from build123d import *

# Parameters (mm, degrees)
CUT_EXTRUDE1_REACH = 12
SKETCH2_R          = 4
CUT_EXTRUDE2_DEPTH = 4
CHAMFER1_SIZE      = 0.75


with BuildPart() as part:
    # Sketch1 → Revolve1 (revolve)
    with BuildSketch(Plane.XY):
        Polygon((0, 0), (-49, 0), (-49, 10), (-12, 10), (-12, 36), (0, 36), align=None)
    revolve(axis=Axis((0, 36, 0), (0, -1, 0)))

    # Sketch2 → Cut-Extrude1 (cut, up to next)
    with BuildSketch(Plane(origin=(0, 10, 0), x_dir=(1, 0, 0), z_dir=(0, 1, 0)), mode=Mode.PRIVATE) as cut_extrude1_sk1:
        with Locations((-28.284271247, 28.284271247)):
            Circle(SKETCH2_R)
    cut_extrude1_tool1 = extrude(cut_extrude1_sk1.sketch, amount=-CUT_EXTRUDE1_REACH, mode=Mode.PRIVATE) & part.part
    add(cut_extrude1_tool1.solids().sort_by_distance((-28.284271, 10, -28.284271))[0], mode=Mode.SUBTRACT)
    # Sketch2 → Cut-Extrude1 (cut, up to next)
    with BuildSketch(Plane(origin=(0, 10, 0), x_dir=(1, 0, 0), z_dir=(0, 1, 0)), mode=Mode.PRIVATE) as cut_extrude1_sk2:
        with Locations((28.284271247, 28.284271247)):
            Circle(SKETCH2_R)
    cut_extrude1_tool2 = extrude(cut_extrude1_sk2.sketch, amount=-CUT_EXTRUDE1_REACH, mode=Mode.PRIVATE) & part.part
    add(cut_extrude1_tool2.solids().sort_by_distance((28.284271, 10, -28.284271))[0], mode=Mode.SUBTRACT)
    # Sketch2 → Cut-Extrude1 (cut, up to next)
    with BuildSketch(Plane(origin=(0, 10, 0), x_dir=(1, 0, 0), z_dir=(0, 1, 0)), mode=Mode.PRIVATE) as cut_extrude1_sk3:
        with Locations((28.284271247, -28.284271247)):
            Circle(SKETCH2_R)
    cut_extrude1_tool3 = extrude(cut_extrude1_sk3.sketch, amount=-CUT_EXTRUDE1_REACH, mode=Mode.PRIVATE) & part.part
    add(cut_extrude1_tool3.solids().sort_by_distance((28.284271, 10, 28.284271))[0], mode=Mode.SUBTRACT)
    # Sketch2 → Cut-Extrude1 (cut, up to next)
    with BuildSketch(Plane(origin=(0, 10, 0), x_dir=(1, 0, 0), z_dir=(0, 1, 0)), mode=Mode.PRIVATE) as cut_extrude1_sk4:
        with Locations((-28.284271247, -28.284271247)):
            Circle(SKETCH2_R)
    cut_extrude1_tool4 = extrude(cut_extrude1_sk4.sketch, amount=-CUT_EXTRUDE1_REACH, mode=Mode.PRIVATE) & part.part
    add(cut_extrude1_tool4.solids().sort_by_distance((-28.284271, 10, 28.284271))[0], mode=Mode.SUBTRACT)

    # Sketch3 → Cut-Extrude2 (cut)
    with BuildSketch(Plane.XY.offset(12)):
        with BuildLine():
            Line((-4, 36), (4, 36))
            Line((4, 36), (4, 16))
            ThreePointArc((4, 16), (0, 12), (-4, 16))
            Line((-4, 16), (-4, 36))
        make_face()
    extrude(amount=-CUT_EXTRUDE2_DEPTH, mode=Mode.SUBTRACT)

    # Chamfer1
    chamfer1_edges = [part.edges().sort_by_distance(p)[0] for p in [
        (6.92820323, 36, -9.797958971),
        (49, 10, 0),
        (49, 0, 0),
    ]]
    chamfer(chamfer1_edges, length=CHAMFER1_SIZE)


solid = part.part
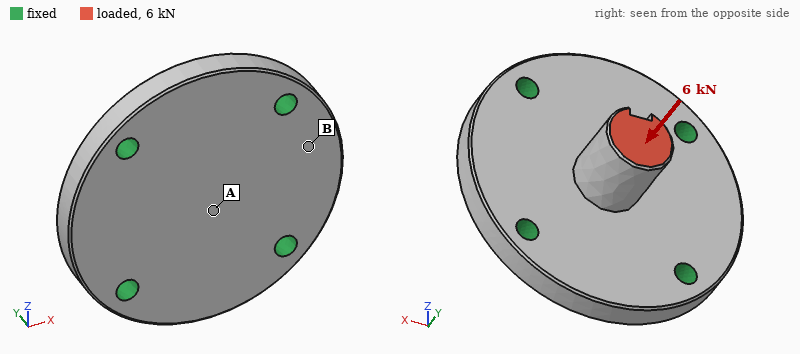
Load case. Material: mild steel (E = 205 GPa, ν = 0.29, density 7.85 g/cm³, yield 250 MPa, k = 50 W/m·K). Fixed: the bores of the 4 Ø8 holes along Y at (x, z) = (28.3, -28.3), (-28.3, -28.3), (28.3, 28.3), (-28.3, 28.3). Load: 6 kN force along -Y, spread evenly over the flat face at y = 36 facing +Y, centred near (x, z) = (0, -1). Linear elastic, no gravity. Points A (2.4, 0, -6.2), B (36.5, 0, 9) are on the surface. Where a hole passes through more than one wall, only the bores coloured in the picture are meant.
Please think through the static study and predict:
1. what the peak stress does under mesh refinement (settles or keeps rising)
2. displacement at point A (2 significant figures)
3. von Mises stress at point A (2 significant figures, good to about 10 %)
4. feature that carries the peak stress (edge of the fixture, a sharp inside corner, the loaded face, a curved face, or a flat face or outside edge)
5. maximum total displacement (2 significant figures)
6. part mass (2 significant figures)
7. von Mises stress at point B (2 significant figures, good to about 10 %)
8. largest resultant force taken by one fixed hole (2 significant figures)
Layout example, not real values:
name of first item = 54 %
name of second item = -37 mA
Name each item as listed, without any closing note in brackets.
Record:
what the peak stress does under mesh refinement = keeps rising
displacement at point A = 9.5 µm
von Mises stress at point A = 28 MPa
feature that carries the peak stress = edge of the fixture
maximum total displacement = 11 µm
part mass = 660 g
von Mises stress at point B = 10 MPa
largest resultant force taken by one fixed hole = 1.6 kN
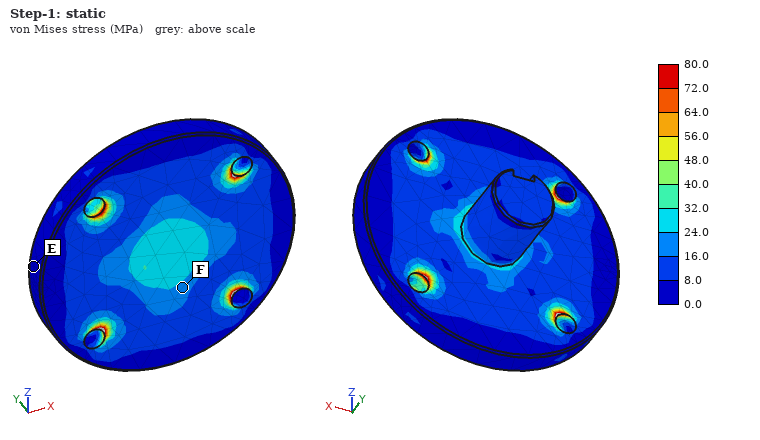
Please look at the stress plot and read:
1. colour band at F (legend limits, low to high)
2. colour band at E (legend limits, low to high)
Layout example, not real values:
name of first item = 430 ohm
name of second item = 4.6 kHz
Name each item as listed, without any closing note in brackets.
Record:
colour band at F = 16.0 to 24.0 MPa
colour band at E = 0.0 to 8.0 MPa
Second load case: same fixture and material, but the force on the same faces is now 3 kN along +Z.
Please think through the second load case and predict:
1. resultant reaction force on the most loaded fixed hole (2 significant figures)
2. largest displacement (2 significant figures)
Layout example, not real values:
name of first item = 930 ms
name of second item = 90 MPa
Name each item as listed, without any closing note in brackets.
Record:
resultant reaction force on the most loaded fixed hole = 1.3 kN
largest displacement = 24 µm
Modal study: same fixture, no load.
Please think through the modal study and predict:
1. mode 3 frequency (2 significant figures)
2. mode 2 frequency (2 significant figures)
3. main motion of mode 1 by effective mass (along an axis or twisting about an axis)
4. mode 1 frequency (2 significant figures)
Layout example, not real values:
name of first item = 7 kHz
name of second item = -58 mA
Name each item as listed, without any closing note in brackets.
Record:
mode 3 frequency = 9700 Hz
mode 2 frequency = 9700 Hz
main motion of mode 1 by effective mass = along Y
mode 1 frequency = 8900 Hz
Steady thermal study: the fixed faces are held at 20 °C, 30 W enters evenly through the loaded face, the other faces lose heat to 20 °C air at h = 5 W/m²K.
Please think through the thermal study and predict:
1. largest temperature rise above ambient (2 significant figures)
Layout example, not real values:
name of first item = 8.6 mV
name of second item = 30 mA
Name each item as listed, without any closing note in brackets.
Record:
largest temperature rise above ambient = 56 K
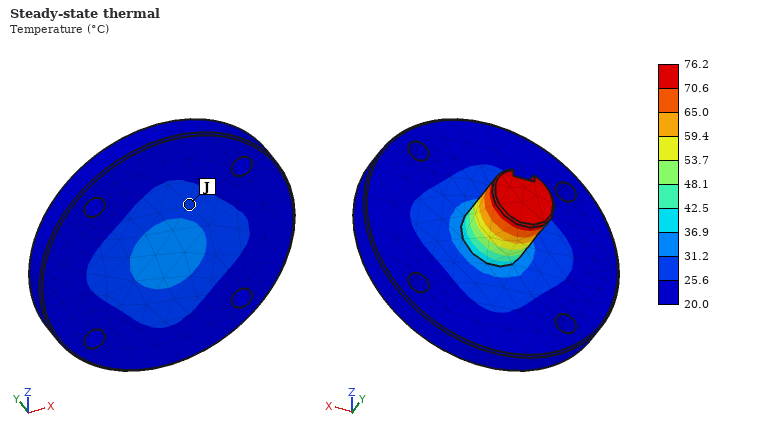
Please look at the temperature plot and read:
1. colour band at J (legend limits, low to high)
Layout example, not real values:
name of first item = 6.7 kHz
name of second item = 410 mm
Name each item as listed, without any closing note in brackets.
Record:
colour band at J = 25.6 to 31.2 °C
